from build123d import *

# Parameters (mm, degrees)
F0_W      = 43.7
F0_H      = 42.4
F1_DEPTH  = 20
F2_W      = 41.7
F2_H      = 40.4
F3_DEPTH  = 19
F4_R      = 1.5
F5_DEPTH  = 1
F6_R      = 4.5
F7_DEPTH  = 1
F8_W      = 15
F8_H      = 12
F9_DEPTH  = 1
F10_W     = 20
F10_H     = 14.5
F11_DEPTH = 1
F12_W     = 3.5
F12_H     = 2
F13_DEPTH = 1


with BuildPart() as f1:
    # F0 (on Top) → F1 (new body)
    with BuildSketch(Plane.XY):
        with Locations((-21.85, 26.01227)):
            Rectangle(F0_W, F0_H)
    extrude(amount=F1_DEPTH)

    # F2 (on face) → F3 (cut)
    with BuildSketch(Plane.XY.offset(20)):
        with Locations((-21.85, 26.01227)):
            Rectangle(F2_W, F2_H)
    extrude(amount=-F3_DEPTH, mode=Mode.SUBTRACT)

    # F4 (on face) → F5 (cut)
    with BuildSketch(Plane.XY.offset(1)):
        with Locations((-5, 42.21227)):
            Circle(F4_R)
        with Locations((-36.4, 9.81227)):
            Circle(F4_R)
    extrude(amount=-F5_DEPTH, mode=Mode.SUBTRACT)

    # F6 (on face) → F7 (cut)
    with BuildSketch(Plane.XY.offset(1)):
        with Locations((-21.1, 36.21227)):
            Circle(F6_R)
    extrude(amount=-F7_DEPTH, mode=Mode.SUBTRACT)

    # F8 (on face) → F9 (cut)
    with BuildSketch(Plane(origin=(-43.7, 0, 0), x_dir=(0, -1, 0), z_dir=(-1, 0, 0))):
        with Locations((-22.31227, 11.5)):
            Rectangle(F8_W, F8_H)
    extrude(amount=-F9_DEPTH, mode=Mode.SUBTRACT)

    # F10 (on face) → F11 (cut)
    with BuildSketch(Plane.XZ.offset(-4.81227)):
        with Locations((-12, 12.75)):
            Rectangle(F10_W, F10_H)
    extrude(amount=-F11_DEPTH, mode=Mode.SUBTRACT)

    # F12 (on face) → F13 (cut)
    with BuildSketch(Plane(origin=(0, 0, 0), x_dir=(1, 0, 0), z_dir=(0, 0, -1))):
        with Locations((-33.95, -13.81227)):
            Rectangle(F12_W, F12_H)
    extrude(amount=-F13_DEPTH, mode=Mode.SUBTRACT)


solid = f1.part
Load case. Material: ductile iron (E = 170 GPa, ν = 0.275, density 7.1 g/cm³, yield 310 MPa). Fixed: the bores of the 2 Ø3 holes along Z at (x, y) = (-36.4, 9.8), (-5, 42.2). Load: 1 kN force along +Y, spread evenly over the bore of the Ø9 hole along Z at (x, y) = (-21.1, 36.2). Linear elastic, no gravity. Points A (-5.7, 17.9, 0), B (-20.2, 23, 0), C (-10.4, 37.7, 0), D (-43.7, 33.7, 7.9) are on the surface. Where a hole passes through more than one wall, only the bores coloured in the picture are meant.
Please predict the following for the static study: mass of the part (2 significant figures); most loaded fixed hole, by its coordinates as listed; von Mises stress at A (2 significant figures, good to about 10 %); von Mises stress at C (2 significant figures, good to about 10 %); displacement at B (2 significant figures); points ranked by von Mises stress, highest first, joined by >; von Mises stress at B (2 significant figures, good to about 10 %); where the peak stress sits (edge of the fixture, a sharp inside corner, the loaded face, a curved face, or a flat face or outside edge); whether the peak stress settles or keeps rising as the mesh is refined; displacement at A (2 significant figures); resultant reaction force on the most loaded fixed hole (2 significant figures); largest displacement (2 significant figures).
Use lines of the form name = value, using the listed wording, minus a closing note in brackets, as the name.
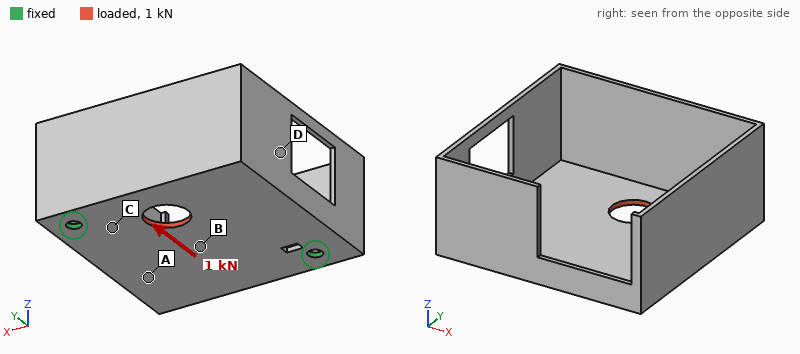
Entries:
mass of the part = 32 g
most loaded fixed hole, by its coordinates as listed = (-5, 42.2)
von Mises stress at A = 12 MPa
von Mises stress at C = 38 MPa
displacement at B = 4.6 µm
points ranked by von Mises stress, highest first, joined by > = C > B > A > D
von Mises stress at B = 22 MPa
where the peak stress sits = edge of the fixture
whether the peak stress settles or keeps rising as the mesh is refined = keeps rising
displacement at A = 3.7 µm
resultant reaction force on the most loaded fixed hole = 530 N
largest displacement = 8.6 µm
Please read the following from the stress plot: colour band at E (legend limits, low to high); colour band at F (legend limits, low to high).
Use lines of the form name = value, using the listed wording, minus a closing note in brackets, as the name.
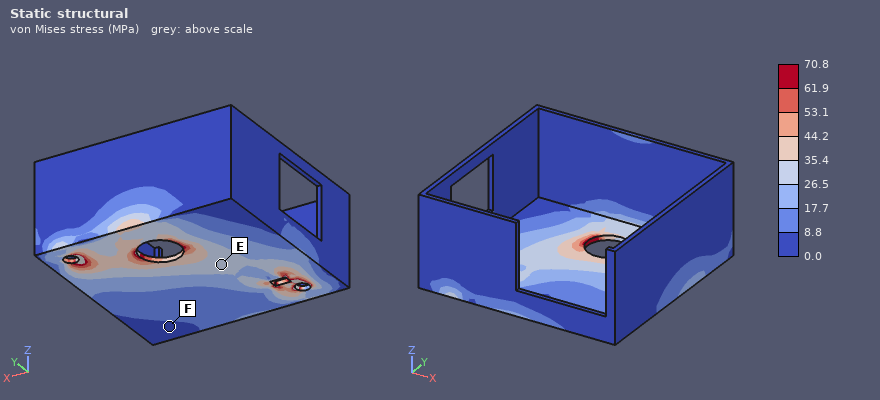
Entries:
colour band at E = 26.5 to 35.4 MPa
colour band at F = 0.0 to 8.8 MPa
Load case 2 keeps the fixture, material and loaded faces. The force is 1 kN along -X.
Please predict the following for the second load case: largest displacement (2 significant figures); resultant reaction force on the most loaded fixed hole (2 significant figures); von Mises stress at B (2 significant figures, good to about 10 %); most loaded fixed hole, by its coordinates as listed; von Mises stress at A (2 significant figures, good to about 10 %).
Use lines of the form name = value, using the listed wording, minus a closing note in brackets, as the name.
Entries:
largest displacement = 6.9 µm
resultant reaction force on the most loaded fixed hole = 730 N
von Mises stress at B = 10 MPa
most loaded fixed hole, by its coordinates as listed = (-5, 42.2)
von Mises stress at A = 12 MPa
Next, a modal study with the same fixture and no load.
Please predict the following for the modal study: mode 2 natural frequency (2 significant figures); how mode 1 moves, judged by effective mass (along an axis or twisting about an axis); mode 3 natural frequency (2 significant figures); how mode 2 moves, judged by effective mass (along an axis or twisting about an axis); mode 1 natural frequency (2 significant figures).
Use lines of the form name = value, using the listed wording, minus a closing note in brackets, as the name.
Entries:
mode 2 natural frequency = 1300 Hz
how mode 1 moves, judged by effective mass = along Z
mode 3 natural frequency = 2600 Hz
how mode 2 moves, judged by effective mass = along Z
mode 1 natural frequency = 990 Hz
